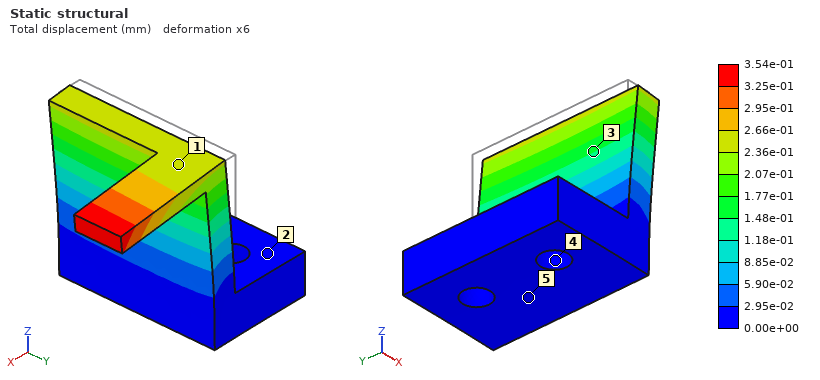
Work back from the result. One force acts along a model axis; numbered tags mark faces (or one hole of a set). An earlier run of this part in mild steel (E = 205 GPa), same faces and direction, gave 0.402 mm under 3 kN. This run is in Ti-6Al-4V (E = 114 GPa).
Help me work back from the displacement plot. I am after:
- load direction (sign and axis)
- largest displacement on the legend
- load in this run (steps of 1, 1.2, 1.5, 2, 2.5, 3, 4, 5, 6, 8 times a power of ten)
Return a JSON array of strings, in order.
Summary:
["+X", "3.54e-01 mm", "1.5 kN"]
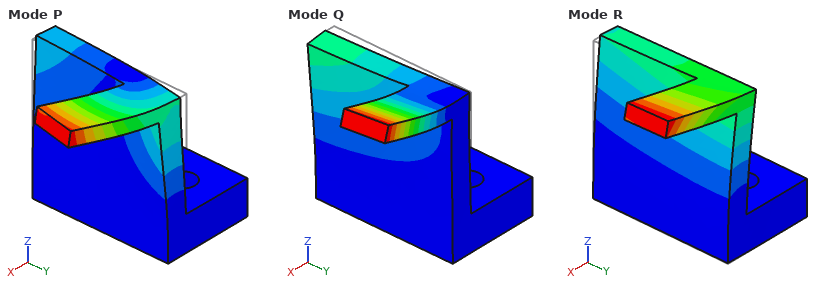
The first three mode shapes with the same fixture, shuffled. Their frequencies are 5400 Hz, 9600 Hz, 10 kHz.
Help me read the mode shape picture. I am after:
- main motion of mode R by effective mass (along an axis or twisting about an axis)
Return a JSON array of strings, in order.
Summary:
["along X"]
